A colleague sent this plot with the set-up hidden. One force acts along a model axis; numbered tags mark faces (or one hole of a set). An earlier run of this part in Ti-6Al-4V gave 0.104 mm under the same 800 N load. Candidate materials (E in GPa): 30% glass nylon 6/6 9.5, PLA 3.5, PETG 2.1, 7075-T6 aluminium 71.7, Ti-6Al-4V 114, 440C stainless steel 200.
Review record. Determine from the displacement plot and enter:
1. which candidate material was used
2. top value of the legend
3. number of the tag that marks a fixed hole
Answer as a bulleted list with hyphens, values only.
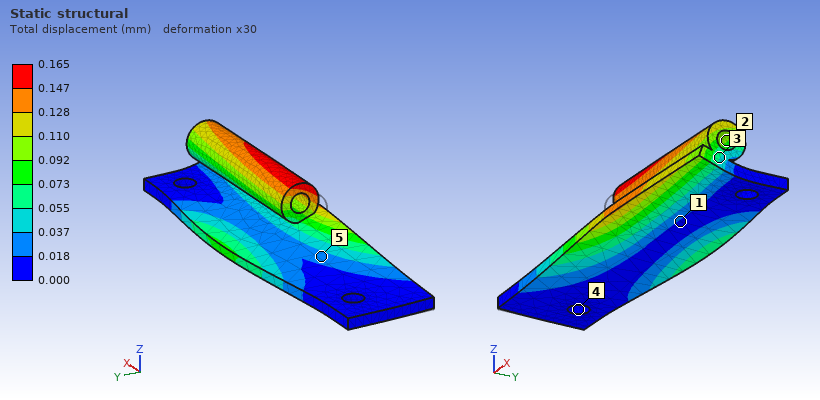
- 7075-T6 aluminium
- 0.165 mm
- 4
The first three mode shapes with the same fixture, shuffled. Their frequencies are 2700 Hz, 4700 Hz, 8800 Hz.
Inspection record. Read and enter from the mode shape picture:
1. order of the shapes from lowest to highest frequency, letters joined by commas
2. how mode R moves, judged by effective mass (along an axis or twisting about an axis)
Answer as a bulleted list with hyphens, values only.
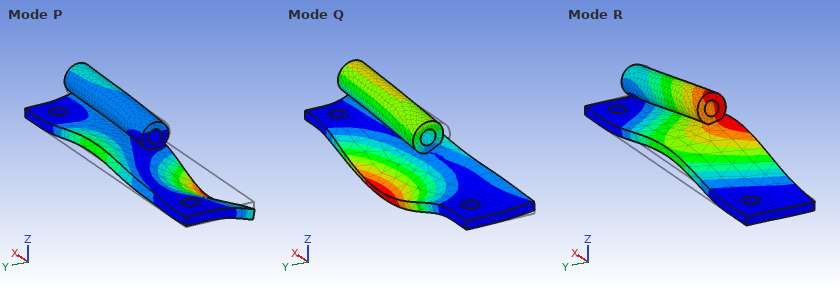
- R, Q, P
- along Z
